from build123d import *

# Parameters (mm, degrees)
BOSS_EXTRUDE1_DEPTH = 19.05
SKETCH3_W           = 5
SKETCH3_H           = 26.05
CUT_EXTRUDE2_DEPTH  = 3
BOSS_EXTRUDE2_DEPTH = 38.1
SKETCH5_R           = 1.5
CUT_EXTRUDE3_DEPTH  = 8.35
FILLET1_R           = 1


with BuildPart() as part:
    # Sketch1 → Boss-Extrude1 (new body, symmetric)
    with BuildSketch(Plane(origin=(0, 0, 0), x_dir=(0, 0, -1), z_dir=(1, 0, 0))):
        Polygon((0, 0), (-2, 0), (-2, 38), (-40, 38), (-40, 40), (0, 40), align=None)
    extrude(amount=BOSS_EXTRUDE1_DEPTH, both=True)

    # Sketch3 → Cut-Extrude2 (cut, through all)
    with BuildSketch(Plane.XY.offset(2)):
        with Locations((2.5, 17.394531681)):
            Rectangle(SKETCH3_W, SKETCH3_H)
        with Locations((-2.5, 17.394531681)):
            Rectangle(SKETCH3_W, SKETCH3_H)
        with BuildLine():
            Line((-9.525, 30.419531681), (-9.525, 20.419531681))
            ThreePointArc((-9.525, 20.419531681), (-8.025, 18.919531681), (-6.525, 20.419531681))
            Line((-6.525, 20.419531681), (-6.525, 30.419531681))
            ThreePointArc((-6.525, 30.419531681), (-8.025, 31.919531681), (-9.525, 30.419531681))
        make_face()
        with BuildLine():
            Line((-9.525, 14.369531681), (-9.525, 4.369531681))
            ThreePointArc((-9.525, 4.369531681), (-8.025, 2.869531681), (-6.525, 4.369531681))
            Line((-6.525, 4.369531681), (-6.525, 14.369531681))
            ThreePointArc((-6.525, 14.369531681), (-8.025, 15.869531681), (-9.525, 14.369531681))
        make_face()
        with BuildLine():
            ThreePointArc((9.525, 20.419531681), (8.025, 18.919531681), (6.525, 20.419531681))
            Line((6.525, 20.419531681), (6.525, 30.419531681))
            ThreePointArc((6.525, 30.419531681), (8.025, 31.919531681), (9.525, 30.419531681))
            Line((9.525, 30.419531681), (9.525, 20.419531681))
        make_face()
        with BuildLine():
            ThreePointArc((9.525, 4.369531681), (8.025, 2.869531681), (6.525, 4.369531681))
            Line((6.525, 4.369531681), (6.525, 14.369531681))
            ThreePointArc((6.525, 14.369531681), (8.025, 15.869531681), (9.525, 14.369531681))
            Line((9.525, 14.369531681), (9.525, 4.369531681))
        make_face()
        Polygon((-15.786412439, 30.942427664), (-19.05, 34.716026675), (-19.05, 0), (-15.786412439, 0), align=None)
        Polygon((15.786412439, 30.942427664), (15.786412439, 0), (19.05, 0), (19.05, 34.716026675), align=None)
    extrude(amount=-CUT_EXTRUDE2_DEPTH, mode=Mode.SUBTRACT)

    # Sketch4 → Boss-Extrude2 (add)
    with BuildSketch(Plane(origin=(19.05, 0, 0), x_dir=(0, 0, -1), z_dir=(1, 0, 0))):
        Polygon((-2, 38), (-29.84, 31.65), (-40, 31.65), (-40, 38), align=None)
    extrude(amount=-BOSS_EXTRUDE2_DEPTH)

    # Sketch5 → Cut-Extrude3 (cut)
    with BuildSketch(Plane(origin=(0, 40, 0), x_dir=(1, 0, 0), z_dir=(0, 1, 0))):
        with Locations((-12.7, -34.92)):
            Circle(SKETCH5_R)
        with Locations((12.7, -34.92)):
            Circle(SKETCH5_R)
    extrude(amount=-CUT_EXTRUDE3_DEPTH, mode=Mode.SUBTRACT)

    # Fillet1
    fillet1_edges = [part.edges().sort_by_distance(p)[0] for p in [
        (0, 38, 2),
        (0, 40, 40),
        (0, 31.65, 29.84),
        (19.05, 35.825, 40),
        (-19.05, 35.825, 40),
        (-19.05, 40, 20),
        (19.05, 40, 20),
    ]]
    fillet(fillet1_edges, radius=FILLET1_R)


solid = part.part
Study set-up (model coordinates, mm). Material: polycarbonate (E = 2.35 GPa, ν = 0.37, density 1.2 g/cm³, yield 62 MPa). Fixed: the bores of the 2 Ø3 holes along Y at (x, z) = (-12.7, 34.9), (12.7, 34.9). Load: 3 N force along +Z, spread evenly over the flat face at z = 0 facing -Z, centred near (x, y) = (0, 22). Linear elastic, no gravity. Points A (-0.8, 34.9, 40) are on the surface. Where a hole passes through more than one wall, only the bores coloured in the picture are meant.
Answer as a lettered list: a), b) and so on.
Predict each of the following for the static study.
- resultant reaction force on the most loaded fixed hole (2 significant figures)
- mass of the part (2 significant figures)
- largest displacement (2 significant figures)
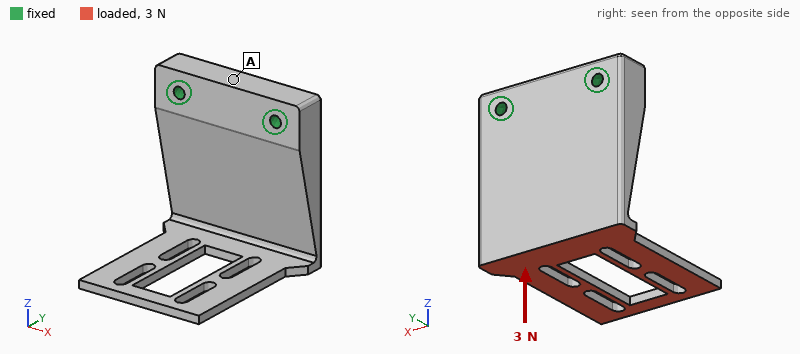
a) 1.5 N
b) 12 g
c) 0.65 mm
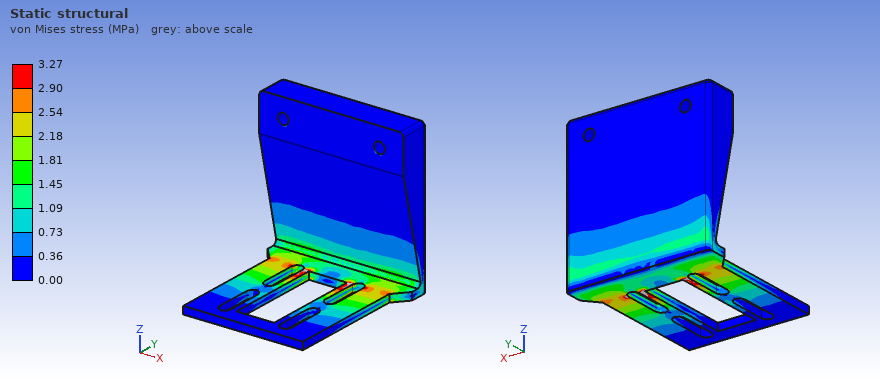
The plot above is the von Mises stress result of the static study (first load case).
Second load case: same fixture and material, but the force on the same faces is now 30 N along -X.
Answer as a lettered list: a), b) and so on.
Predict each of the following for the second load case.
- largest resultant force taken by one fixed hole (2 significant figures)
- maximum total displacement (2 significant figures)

a) 44 N
b) 0.66 mm
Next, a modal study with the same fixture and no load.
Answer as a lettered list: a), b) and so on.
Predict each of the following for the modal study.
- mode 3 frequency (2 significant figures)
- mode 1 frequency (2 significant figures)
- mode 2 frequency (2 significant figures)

a) 840 Hz
b) 280 Hz
c) 640 Hz
